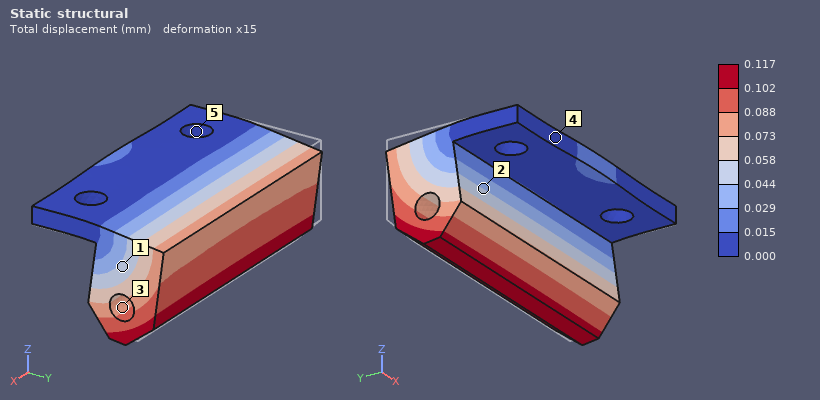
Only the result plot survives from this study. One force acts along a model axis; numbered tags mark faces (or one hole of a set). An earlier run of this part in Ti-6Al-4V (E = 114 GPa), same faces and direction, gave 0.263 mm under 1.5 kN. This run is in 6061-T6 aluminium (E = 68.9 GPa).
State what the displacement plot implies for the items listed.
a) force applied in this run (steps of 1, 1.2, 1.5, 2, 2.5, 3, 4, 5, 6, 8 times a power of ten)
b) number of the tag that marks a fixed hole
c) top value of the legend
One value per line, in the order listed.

400 N
5
0.117 mm
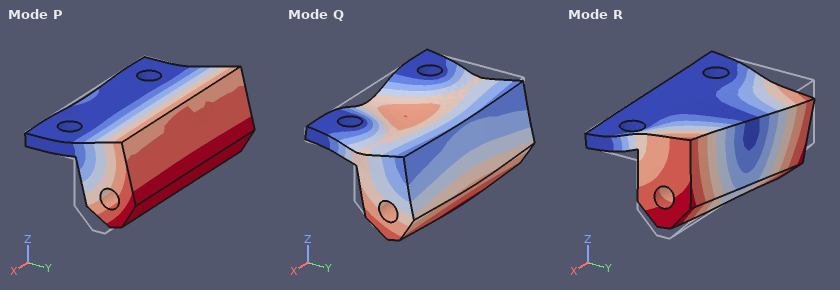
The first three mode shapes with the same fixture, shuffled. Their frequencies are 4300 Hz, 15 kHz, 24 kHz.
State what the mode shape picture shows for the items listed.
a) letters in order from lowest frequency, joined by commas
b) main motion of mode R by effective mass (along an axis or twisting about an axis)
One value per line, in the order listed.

P, R, Q
along X
